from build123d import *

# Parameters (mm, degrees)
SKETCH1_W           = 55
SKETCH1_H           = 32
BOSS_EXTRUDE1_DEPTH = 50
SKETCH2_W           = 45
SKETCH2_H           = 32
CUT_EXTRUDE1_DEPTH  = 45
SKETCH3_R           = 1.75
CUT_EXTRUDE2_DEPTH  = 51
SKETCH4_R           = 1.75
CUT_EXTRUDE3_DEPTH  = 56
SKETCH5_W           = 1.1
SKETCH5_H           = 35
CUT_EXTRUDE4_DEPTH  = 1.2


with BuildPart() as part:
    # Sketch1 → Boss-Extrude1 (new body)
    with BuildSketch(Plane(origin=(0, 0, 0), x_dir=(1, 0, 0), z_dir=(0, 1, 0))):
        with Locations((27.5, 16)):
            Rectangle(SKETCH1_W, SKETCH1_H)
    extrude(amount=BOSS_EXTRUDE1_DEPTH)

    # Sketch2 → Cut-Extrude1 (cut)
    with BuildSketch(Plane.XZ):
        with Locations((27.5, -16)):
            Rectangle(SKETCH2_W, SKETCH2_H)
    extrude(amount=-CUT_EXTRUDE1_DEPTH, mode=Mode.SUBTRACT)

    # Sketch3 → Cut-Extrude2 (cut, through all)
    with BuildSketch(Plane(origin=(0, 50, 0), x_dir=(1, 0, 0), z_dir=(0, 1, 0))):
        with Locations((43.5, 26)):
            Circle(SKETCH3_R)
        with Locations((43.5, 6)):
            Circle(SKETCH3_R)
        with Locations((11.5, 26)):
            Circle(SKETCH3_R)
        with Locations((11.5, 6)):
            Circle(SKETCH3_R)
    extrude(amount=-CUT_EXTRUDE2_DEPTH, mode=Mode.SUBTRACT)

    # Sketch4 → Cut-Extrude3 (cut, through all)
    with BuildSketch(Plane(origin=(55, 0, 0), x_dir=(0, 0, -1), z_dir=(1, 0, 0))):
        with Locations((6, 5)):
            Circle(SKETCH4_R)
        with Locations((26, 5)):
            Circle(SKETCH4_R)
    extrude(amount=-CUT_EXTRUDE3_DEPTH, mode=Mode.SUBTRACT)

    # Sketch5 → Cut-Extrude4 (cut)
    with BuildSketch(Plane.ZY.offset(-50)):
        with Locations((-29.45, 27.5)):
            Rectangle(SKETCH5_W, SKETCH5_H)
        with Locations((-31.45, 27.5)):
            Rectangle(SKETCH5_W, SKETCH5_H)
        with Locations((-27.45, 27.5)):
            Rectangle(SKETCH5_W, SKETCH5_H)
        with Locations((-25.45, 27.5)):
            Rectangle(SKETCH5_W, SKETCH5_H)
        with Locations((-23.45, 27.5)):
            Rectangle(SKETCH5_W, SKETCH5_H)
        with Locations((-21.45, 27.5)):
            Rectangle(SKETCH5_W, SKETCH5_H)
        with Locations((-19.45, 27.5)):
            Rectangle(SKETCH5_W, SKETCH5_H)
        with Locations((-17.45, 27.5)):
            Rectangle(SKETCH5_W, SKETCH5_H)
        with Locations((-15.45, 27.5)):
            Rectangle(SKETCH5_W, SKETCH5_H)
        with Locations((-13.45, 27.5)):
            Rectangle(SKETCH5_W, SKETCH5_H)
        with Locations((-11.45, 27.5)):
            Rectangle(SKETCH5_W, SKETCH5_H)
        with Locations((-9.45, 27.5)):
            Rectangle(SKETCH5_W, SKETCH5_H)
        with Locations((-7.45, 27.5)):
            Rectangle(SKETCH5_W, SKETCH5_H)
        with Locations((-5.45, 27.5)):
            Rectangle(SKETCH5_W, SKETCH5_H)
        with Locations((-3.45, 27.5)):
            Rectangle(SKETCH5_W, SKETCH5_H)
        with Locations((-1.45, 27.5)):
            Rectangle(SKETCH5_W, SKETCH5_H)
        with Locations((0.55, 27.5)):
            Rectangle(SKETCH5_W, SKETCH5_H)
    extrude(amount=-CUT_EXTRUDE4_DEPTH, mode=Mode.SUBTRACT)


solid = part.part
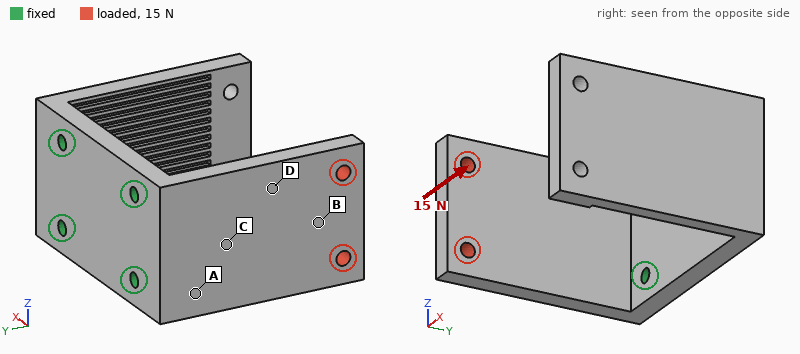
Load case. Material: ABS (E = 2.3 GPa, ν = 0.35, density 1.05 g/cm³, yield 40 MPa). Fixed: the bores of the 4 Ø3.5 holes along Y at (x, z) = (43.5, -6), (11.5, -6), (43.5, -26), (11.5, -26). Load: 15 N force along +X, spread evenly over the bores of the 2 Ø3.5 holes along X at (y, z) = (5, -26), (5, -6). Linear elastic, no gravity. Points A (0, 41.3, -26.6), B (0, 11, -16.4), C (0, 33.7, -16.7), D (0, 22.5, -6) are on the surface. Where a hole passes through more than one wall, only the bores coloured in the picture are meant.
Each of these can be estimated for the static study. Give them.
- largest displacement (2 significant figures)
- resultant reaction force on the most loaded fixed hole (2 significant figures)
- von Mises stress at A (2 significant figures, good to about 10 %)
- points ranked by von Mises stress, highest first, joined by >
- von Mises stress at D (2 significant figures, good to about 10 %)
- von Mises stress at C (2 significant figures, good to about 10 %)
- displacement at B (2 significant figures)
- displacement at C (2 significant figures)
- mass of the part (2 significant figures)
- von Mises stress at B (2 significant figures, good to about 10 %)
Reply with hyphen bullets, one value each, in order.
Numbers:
- 0.85 mm
- 8.4 N
- 3.6 MPa
- A > C > D > B
- 1.9 MPa
- 2.8 MPa
- 0.60 mm
- 0.17 mm
- 23 g
- 0.68 MPa
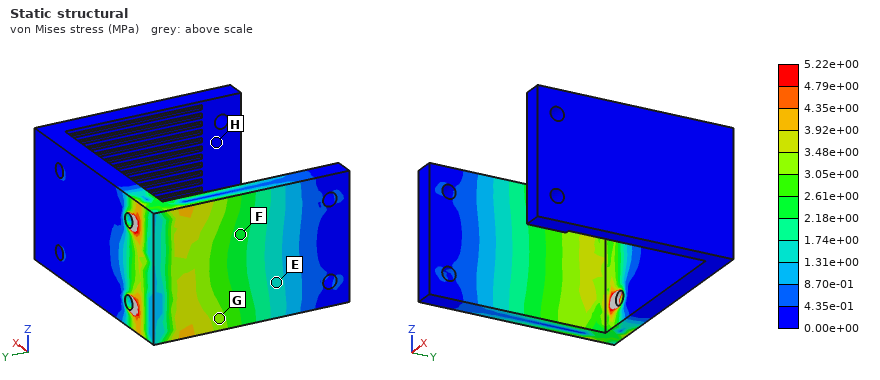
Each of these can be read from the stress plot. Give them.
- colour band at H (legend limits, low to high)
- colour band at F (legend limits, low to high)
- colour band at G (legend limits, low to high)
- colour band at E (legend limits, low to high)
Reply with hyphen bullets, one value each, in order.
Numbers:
- 0.00e+00 to 4.35e-01 MPa
- 2.18e+00 to 2.61e+00 MPa
- 3.05e+00 to 3.48e+00 MPa
- 1.31e+00 to 1.74e+00 MPa
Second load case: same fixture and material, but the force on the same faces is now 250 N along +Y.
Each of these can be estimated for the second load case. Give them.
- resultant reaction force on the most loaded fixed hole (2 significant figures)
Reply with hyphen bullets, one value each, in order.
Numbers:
- 130 N
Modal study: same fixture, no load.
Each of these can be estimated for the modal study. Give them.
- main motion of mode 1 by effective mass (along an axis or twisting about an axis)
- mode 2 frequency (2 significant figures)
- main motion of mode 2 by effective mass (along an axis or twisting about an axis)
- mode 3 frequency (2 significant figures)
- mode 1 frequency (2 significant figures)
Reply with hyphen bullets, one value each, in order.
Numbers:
- along X
- 430 Hz
- along X
- 1100 Hz
- 400 Hz
